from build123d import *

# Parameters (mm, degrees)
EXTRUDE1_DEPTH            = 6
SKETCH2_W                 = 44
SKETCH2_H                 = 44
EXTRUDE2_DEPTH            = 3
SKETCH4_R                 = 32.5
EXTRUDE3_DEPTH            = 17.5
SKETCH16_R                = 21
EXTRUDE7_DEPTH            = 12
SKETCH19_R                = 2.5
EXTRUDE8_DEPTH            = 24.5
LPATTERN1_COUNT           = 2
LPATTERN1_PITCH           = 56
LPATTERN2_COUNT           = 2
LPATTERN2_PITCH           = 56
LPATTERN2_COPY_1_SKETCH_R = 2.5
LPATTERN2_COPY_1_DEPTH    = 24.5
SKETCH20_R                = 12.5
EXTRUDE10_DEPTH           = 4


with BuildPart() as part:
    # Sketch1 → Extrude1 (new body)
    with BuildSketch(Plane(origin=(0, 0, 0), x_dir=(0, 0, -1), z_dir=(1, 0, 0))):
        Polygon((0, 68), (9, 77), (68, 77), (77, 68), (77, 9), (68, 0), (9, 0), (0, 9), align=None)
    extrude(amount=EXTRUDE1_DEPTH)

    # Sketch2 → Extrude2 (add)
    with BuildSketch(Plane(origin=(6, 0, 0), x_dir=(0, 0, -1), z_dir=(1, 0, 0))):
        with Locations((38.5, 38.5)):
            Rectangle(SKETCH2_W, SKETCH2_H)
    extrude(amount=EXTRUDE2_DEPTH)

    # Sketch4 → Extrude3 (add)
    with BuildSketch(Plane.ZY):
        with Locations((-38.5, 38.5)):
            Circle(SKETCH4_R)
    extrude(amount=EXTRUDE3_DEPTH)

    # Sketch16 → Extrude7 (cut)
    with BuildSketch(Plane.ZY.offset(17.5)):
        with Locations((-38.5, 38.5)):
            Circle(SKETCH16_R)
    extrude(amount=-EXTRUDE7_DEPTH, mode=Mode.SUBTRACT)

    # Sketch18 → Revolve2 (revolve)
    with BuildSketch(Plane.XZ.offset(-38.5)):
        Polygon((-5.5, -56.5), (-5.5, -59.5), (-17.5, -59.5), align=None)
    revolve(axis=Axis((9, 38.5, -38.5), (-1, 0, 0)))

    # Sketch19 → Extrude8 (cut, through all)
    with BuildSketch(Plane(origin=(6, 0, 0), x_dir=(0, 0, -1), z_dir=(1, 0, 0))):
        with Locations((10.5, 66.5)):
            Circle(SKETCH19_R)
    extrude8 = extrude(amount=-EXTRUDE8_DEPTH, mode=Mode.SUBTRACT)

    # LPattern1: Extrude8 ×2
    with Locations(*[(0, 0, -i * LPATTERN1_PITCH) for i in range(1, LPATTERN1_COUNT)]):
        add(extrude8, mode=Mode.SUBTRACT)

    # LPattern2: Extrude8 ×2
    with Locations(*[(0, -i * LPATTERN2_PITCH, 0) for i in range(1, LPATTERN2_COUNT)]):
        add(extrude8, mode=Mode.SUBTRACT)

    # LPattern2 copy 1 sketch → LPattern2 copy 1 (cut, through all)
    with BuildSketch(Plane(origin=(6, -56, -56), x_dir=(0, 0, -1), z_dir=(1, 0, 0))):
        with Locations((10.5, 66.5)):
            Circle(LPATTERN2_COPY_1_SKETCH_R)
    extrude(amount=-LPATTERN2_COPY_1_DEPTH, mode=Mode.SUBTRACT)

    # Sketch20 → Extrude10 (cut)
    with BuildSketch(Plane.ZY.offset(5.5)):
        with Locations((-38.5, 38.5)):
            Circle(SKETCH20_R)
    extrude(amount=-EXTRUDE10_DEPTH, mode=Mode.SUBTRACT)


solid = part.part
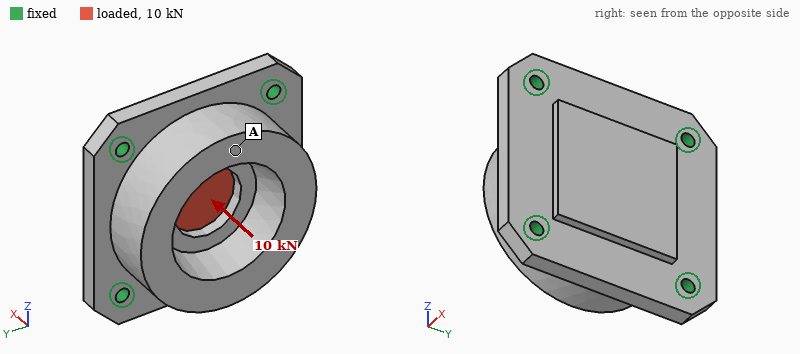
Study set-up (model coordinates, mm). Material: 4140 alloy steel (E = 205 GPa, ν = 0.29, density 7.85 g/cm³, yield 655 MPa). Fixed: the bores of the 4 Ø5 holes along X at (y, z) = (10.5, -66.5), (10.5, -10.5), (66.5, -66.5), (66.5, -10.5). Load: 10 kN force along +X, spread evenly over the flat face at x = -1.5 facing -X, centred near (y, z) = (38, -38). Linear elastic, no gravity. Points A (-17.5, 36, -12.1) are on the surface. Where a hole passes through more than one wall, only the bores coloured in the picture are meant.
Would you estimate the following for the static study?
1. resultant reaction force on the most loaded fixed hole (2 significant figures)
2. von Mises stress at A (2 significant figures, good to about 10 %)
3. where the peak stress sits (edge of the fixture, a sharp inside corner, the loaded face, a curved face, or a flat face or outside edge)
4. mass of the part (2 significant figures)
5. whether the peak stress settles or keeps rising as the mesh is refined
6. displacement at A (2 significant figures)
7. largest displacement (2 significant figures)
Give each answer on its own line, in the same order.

2.7 kN
18 MPa
edge of the fixture
640 g
keeps rising
7.2 µm
13 µm
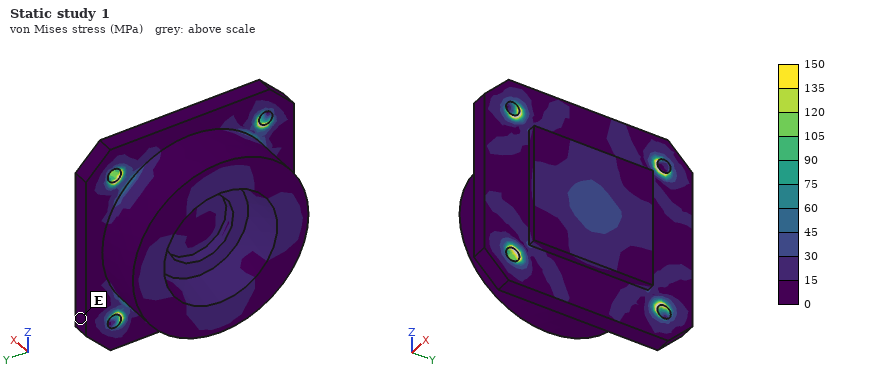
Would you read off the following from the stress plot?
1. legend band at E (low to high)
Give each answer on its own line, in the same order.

0 to 15 MPa
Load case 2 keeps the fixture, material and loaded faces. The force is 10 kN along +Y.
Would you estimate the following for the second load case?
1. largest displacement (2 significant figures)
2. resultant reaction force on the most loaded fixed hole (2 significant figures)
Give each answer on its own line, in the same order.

4.7 µm
2.7 kN
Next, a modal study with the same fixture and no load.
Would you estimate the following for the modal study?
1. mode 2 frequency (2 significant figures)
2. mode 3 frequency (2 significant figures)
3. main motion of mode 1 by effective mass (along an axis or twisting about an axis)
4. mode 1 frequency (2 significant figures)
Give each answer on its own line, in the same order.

10 kHz
10 kHz
along X
8200 Hz
